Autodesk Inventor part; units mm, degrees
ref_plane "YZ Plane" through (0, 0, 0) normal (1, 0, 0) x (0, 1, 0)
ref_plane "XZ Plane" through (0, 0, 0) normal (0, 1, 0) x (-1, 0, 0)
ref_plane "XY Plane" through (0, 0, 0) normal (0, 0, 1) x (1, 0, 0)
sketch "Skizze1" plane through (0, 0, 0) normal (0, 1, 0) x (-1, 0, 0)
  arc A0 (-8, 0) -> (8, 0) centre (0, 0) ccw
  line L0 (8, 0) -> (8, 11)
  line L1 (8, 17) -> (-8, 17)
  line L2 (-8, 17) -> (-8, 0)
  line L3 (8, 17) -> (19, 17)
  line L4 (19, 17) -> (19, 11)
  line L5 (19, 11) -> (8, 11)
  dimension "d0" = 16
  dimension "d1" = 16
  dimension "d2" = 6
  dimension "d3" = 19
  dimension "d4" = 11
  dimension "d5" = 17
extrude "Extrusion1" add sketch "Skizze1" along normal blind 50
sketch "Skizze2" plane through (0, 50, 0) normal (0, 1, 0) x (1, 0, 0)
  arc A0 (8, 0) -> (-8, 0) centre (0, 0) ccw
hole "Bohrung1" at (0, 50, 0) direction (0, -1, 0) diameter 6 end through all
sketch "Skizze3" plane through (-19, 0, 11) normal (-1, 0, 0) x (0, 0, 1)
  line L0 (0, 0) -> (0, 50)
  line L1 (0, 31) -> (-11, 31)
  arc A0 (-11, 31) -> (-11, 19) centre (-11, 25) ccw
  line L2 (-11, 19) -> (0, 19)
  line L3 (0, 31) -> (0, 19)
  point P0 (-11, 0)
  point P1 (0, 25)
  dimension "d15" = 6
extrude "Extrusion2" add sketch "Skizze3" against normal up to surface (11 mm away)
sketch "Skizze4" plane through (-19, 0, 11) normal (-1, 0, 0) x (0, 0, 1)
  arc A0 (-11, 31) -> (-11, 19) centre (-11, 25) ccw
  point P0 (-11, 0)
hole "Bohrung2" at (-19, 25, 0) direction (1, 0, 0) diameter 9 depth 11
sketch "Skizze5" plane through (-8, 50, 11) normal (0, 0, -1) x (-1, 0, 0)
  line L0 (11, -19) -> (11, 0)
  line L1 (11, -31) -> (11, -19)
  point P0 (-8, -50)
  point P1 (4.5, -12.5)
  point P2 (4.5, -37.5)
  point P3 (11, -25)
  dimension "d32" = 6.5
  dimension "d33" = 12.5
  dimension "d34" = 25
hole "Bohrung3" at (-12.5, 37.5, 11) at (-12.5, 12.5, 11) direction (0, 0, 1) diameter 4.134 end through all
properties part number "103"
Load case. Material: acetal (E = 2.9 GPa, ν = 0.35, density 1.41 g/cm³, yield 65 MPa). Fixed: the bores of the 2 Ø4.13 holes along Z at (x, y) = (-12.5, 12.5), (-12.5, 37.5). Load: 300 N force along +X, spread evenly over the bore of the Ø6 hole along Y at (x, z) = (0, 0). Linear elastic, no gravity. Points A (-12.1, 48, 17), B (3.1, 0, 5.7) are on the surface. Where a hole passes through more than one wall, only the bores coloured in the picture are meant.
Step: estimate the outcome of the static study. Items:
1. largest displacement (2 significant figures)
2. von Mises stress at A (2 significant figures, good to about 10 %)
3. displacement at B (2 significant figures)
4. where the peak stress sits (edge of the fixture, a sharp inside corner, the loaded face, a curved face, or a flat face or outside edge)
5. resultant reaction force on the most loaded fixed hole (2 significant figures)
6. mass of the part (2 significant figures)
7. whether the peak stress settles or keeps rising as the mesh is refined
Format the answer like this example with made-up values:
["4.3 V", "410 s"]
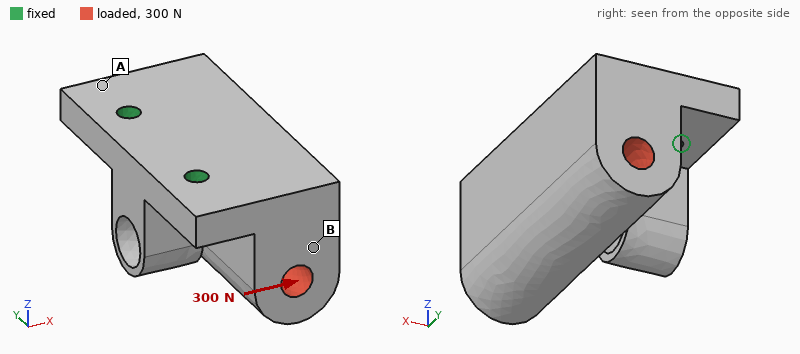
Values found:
["0.27 mm", "4.0 MPa", "0.16 mm", "edge of the fixture", "150 N", "31 g", "keeps rising"]
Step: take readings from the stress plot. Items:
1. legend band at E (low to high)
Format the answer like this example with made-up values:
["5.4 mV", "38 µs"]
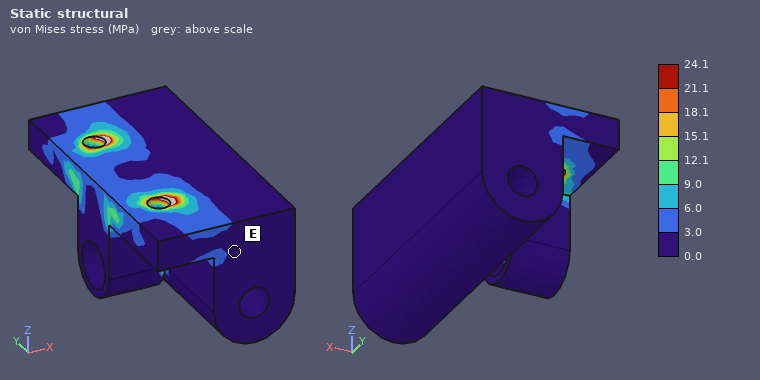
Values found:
["0.0 to 3.0 MPa"]
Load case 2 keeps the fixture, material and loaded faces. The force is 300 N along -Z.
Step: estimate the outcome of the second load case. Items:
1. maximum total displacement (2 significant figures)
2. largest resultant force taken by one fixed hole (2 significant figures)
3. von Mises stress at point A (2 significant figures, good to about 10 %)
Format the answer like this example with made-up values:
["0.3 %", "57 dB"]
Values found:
["0.20 mm", "150 N", "2.8 MPa"]
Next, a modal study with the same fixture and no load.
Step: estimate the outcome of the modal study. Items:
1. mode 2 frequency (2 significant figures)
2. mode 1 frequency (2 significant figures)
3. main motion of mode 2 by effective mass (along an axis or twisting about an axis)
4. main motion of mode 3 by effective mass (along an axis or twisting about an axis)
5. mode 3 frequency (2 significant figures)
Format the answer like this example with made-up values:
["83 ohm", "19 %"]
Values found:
["2900 Hz", "1300 Hz", "along Y", "along Y", "3700 Hz"]
